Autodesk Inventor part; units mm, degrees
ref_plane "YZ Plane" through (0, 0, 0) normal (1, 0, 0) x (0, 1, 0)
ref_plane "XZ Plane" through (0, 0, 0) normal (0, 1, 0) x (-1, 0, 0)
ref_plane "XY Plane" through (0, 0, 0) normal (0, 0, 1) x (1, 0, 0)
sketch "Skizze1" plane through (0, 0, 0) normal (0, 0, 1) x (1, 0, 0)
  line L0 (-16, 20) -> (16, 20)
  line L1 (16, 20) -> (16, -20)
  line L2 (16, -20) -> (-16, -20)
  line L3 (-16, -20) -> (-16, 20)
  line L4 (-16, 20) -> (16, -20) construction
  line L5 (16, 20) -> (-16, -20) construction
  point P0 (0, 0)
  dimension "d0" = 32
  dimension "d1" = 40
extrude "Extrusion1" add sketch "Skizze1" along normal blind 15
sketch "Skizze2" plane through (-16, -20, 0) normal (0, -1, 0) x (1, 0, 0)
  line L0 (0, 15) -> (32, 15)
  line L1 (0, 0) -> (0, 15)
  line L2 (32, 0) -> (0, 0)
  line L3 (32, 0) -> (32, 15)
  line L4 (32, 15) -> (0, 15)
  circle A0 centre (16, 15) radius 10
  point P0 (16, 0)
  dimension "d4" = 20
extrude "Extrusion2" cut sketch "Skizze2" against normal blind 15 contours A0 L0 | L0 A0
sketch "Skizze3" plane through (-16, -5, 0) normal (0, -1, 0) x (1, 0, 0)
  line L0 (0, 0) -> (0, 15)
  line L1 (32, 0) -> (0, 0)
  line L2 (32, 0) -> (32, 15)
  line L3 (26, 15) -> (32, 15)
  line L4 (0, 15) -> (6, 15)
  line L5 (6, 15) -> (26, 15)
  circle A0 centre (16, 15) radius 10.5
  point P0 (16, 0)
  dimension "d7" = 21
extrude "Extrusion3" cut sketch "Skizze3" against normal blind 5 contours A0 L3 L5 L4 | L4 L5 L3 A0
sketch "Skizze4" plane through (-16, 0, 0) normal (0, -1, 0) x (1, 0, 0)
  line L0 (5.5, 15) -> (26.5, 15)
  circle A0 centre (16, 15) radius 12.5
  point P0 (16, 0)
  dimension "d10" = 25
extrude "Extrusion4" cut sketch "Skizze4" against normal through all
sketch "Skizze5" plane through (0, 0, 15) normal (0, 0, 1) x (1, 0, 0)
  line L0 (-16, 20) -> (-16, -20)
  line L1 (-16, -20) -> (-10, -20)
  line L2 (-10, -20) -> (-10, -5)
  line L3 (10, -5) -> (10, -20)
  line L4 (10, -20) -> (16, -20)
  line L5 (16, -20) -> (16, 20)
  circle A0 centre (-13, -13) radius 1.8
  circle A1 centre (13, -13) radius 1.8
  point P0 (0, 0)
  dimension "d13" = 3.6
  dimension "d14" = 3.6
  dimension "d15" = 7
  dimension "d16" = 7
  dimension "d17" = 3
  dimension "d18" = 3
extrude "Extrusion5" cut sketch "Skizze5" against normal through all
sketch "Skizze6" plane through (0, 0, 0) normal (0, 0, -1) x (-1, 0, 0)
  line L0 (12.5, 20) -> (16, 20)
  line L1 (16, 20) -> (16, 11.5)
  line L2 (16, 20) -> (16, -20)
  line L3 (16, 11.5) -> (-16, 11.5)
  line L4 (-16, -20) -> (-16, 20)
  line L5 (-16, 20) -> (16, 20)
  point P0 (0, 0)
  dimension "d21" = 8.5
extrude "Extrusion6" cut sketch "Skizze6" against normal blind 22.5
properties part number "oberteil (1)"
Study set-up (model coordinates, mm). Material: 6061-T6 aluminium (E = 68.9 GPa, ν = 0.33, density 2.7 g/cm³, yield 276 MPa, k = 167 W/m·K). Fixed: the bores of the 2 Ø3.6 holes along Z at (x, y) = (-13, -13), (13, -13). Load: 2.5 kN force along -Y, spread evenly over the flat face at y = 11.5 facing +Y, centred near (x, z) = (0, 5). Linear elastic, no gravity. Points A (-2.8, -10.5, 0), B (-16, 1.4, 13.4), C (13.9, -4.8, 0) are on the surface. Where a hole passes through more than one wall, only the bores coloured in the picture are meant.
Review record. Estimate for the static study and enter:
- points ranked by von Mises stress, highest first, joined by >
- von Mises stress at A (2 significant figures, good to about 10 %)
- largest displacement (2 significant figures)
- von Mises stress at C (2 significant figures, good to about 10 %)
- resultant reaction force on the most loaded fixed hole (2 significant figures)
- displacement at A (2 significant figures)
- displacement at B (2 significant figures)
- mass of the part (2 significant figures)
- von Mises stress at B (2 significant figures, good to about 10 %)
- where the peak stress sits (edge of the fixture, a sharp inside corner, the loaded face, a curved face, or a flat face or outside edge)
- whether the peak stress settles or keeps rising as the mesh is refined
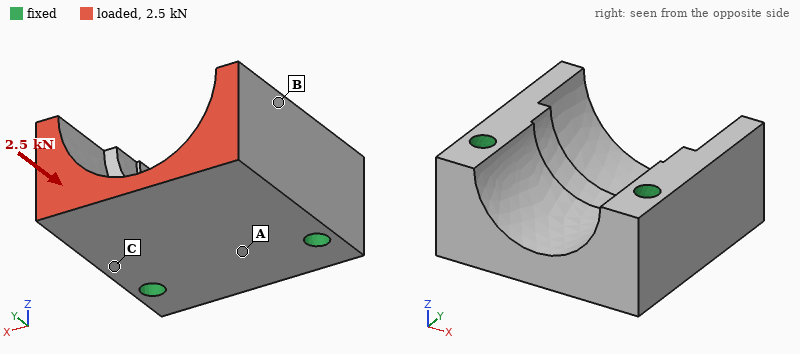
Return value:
C > B > A
3.9 MPa
5.5 µm
14 MPa
1.3 kN
1.9 µm
1.6 µm
24 g
8.6 MPa
edge of the fixture
keeps rising
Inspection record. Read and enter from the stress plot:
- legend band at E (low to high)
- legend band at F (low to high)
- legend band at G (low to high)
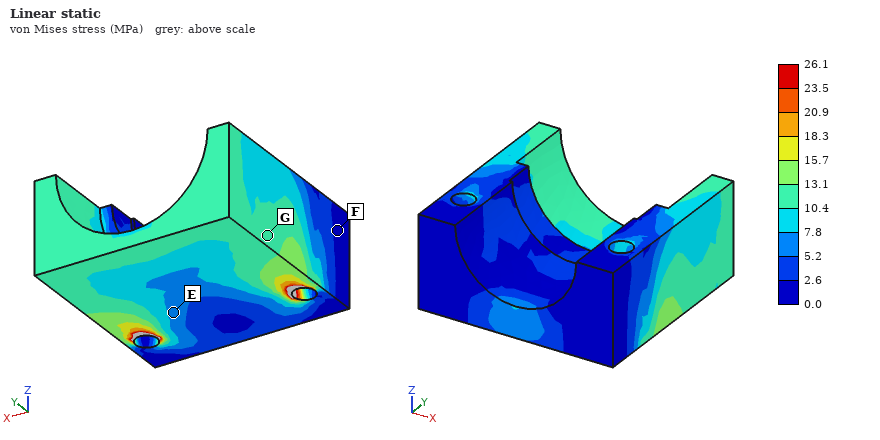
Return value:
5.2 to 7.8 MPa
0.0 to 2.6 MPa
10.4 to 13.1 MPa
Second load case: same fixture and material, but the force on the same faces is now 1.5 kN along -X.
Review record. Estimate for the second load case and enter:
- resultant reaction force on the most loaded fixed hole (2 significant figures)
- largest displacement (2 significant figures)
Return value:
1.5 kN
33 µm
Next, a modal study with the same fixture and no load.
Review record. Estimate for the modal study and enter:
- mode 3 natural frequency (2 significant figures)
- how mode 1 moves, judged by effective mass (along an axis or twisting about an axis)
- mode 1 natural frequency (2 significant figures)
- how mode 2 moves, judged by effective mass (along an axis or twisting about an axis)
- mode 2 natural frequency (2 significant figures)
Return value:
21 kHz
along Z
16 kHz
along X
17 kHz
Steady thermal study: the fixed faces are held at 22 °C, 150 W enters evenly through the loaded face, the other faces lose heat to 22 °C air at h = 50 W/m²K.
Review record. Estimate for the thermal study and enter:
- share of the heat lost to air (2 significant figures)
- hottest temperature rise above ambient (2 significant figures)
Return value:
3.5 %
82 K
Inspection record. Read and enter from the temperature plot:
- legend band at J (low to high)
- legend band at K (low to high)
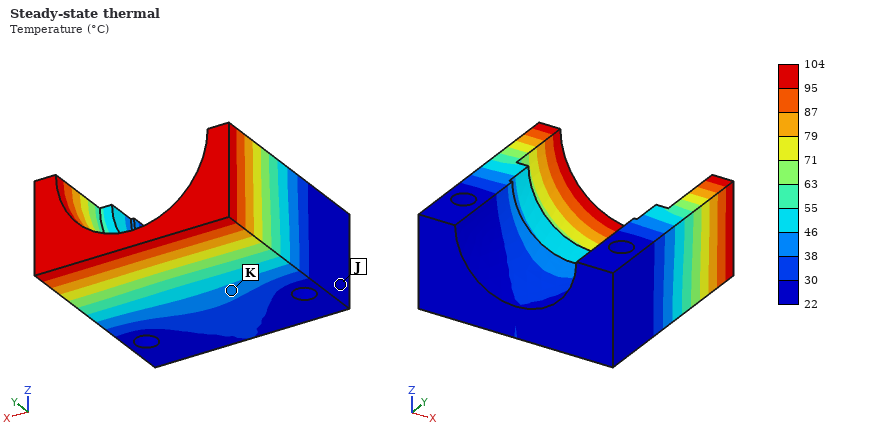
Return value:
22 to 30 °C
38 to 46 °C
